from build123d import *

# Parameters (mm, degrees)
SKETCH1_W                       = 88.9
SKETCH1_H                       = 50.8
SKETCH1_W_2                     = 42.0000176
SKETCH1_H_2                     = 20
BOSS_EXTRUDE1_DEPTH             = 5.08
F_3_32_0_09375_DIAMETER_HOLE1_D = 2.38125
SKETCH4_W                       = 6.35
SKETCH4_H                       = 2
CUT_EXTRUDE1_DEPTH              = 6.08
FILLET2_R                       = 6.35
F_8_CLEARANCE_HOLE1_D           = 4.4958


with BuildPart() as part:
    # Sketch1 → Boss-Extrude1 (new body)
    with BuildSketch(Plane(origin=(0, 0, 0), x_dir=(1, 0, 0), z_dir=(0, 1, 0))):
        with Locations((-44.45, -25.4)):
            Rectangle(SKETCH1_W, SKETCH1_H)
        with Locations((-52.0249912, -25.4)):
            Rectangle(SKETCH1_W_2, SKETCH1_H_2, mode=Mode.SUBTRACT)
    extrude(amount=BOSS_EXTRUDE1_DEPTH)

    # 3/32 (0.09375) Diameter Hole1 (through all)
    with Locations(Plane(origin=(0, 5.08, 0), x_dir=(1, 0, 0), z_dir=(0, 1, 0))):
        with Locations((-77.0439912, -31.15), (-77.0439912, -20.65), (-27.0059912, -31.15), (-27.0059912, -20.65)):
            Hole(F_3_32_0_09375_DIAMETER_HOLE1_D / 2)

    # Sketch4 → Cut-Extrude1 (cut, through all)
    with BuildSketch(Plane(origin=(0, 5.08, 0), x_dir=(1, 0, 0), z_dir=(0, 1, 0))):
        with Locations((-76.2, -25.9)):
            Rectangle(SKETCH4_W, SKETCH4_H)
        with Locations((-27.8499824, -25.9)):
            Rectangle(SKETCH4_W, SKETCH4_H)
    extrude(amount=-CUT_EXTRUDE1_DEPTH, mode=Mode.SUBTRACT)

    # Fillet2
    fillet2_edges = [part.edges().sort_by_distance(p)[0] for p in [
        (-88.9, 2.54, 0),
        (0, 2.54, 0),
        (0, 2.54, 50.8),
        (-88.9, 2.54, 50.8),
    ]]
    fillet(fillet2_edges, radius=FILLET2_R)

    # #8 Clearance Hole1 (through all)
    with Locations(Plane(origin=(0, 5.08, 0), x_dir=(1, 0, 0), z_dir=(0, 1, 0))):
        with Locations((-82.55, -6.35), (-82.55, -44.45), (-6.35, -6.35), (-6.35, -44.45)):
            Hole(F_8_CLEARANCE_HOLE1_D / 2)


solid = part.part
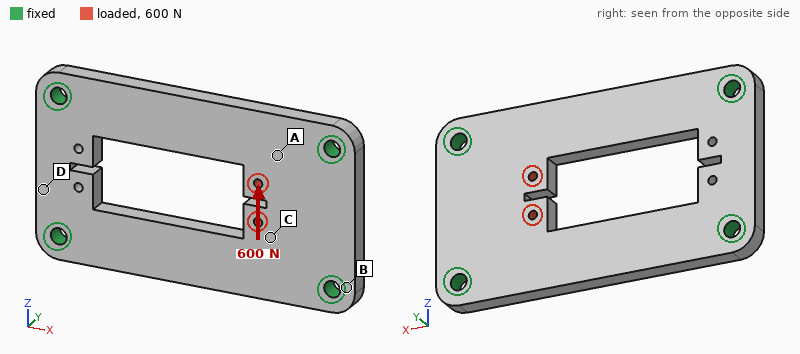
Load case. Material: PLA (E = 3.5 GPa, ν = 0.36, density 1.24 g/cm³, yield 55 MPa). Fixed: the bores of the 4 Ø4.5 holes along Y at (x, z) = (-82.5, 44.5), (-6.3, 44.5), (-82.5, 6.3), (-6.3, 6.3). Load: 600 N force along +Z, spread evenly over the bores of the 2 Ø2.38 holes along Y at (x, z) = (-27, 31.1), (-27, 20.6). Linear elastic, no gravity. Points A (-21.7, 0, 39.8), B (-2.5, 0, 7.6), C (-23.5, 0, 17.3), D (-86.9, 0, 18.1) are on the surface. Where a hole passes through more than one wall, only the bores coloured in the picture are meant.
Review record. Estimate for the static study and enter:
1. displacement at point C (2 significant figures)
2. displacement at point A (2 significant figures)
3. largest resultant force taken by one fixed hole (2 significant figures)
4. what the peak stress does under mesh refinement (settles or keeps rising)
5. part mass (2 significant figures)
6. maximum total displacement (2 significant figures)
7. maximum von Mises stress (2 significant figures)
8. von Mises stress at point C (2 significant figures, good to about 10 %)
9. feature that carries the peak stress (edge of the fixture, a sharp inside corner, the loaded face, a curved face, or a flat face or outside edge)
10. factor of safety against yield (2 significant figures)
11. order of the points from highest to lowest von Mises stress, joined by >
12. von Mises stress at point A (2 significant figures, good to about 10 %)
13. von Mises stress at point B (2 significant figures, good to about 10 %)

41 µm
37 µm
360 N
settles
22 g
61 µm
16 MPa
5.2 MPa
the loaded face
3.4
C > A > B > D
4.3 MPa
2.1 MPa
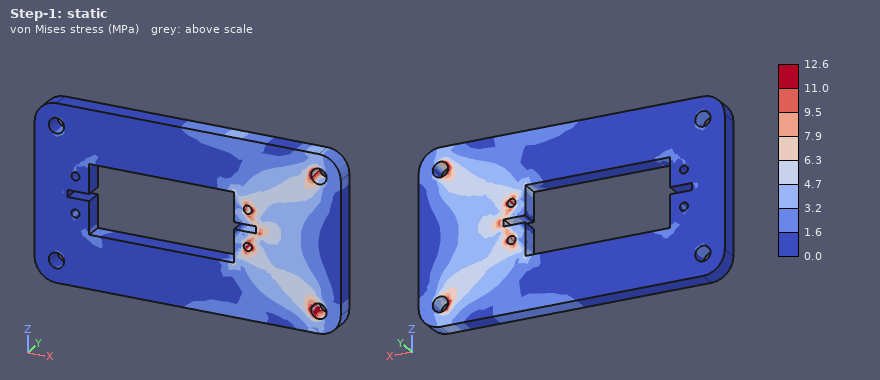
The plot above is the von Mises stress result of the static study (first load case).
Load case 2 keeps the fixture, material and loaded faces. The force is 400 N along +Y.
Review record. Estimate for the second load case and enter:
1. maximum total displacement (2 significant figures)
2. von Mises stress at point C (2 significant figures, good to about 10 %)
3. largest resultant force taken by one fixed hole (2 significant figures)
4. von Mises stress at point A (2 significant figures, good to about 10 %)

0.86 mm
18 MPa
170 N
10 MPa
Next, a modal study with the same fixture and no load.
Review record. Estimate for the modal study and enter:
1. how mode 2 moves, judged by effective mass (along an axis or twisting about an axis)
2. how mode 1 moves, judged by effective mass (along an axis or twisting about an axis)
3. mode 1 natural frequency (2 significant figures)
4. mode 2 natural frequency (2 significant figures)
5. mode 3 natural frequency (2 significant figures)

twisting about X
along Y
1500 Hz
1800 Hz
3400 Hz
